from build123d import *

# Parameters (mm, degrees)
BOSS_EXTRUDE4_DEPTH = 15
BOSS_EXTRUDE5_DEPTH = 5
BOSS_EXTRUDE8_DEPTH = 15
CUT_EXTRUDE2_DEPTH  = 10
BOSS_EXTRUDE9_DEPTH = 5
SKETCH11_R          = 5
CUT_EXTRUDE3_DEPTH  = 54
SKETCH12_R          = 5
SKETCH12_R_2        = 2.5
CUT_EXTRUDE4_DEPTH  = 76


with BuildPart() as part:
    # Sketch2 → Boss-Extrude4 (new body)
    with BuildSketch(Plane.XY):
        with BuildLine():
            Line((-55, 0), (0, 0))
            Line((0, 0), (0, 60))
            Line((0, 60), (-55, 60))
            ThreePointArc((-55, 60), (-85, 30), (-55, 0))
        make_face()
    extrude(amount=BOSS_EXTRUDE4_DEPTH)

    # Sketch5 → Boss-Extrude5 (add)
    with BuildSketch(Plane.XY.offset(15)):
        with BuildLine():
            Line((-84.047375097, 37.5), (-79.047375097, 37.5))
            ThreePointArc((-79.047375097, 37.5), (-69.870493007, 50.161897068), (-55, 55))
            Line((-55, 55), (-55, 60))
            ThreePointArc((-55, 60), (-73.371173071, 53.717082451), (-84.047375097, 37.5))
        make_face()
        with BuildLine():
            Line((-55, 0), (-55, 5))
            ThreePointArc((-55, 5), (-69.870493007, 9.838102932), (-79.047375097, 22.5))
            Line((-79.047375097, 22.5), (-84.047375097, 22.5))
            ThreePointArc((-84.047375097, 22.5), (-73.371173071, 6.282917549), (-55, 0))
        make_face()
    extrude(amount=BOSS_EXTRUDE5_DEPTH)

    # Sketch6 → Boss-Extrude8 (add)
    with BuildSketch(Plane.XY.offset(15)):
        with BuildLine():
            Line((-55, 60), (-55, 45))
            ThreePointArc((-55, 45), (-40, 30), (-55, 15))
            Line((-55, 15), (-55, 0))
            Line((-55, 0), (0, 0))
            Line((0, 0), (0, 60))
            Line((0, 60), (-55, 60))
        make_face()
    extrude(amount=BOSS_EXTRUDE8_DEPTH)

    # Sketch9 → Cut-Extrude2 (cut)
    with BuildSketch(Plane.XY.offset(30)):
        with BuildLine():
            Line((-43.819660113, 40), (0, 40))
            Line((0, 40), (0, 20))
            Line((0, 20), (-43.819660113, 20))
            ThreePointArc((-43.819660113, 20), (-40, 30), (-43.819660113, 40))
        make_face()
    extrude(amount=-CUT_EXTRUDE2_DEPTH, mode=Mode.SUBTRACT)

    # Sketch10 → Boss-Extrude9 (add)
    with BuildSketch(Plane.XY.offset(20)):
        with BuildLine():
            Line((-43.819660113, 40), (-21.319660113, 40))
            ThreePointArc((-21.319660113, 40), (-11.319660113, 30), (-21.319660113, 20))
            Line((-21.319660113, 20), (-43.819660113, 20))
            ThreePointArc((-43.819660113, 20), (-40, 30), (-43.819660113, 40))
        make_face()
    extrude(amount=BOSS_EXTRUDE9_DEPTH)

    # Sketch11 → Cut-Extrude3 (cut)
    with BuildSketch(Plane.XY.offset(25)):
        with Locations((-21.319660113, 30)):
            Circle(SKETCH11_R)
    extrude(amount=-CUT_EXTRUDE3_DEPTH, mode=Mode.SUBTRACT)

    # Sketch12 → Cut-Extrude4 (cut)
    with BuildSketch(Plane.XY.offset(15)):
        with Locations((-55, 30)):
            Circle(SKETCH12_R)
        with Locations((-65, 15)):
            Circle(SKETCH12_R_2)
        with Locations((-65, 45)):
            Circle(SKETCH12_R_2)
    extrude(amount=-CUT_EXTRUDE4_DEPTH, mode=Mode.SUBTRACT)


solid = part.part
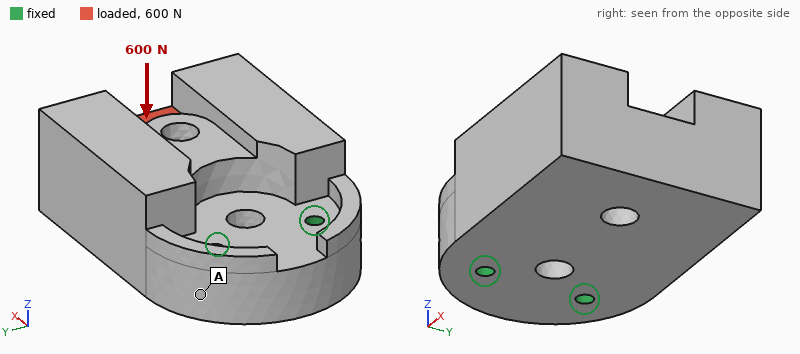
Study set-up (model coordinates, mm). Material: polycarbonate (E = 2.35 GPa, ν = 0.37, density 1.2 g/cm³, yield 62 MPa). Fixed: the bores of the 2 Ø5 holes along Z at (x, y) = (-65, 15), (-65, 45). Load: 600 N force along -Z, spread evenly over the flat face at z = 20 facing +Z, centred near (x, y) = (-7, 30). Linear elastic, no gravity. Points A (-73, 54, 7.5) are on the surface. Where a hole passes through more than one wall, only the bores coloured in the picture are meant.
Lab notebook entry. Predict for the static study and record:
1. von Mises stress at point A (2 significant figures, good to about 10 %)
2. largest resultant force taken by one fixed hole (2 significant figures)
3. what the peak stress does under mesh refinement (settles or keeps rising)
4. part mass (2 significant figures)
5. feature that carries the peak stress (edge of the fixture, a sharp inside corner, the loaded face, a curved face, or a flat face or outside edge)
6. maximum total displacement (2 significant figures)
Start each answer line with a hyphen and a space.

- 5.5 MPa
- 300 N
- keeps rising
- 130 g
- edge of the fixture
- 1.1 mm
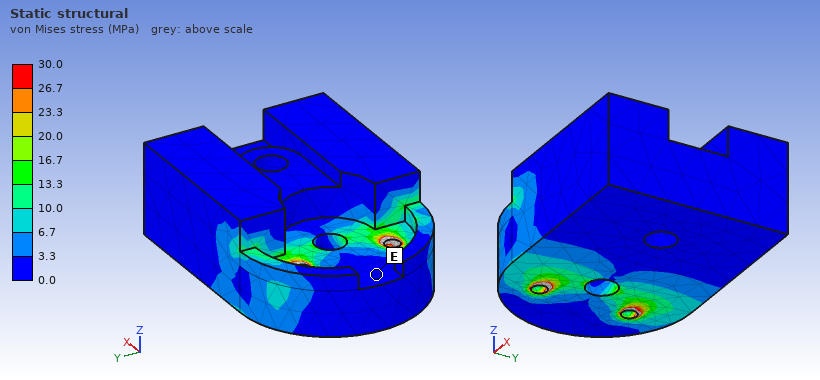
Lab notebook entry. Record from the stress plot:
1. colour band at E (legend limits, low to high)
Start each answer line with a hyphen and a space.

- 0.0 to 3.3 MPa
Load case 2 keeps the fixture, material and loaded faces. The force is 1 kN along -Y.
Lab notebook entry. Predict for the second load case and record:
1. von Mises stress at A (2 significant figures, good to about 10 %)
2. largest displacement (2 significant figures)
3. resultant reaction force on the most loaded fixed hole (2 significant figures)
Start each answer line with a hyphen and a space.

- 4.4 MPa
- 0.38 mm
- 1.8 kN
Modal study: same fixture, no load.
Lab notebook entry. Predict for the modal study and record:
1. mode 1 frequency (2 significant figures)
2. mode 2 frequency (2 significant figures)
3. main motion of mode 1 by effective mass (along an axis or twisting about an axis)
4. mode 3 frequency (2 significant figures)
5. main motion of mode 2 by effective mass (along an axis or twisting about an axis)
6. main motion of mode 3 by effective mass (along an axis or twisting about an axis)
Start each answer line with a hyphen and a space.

- 570 Hz
- 1200 Hz
- along Z
- 1500 Hz
- along Y
- twisting about X
